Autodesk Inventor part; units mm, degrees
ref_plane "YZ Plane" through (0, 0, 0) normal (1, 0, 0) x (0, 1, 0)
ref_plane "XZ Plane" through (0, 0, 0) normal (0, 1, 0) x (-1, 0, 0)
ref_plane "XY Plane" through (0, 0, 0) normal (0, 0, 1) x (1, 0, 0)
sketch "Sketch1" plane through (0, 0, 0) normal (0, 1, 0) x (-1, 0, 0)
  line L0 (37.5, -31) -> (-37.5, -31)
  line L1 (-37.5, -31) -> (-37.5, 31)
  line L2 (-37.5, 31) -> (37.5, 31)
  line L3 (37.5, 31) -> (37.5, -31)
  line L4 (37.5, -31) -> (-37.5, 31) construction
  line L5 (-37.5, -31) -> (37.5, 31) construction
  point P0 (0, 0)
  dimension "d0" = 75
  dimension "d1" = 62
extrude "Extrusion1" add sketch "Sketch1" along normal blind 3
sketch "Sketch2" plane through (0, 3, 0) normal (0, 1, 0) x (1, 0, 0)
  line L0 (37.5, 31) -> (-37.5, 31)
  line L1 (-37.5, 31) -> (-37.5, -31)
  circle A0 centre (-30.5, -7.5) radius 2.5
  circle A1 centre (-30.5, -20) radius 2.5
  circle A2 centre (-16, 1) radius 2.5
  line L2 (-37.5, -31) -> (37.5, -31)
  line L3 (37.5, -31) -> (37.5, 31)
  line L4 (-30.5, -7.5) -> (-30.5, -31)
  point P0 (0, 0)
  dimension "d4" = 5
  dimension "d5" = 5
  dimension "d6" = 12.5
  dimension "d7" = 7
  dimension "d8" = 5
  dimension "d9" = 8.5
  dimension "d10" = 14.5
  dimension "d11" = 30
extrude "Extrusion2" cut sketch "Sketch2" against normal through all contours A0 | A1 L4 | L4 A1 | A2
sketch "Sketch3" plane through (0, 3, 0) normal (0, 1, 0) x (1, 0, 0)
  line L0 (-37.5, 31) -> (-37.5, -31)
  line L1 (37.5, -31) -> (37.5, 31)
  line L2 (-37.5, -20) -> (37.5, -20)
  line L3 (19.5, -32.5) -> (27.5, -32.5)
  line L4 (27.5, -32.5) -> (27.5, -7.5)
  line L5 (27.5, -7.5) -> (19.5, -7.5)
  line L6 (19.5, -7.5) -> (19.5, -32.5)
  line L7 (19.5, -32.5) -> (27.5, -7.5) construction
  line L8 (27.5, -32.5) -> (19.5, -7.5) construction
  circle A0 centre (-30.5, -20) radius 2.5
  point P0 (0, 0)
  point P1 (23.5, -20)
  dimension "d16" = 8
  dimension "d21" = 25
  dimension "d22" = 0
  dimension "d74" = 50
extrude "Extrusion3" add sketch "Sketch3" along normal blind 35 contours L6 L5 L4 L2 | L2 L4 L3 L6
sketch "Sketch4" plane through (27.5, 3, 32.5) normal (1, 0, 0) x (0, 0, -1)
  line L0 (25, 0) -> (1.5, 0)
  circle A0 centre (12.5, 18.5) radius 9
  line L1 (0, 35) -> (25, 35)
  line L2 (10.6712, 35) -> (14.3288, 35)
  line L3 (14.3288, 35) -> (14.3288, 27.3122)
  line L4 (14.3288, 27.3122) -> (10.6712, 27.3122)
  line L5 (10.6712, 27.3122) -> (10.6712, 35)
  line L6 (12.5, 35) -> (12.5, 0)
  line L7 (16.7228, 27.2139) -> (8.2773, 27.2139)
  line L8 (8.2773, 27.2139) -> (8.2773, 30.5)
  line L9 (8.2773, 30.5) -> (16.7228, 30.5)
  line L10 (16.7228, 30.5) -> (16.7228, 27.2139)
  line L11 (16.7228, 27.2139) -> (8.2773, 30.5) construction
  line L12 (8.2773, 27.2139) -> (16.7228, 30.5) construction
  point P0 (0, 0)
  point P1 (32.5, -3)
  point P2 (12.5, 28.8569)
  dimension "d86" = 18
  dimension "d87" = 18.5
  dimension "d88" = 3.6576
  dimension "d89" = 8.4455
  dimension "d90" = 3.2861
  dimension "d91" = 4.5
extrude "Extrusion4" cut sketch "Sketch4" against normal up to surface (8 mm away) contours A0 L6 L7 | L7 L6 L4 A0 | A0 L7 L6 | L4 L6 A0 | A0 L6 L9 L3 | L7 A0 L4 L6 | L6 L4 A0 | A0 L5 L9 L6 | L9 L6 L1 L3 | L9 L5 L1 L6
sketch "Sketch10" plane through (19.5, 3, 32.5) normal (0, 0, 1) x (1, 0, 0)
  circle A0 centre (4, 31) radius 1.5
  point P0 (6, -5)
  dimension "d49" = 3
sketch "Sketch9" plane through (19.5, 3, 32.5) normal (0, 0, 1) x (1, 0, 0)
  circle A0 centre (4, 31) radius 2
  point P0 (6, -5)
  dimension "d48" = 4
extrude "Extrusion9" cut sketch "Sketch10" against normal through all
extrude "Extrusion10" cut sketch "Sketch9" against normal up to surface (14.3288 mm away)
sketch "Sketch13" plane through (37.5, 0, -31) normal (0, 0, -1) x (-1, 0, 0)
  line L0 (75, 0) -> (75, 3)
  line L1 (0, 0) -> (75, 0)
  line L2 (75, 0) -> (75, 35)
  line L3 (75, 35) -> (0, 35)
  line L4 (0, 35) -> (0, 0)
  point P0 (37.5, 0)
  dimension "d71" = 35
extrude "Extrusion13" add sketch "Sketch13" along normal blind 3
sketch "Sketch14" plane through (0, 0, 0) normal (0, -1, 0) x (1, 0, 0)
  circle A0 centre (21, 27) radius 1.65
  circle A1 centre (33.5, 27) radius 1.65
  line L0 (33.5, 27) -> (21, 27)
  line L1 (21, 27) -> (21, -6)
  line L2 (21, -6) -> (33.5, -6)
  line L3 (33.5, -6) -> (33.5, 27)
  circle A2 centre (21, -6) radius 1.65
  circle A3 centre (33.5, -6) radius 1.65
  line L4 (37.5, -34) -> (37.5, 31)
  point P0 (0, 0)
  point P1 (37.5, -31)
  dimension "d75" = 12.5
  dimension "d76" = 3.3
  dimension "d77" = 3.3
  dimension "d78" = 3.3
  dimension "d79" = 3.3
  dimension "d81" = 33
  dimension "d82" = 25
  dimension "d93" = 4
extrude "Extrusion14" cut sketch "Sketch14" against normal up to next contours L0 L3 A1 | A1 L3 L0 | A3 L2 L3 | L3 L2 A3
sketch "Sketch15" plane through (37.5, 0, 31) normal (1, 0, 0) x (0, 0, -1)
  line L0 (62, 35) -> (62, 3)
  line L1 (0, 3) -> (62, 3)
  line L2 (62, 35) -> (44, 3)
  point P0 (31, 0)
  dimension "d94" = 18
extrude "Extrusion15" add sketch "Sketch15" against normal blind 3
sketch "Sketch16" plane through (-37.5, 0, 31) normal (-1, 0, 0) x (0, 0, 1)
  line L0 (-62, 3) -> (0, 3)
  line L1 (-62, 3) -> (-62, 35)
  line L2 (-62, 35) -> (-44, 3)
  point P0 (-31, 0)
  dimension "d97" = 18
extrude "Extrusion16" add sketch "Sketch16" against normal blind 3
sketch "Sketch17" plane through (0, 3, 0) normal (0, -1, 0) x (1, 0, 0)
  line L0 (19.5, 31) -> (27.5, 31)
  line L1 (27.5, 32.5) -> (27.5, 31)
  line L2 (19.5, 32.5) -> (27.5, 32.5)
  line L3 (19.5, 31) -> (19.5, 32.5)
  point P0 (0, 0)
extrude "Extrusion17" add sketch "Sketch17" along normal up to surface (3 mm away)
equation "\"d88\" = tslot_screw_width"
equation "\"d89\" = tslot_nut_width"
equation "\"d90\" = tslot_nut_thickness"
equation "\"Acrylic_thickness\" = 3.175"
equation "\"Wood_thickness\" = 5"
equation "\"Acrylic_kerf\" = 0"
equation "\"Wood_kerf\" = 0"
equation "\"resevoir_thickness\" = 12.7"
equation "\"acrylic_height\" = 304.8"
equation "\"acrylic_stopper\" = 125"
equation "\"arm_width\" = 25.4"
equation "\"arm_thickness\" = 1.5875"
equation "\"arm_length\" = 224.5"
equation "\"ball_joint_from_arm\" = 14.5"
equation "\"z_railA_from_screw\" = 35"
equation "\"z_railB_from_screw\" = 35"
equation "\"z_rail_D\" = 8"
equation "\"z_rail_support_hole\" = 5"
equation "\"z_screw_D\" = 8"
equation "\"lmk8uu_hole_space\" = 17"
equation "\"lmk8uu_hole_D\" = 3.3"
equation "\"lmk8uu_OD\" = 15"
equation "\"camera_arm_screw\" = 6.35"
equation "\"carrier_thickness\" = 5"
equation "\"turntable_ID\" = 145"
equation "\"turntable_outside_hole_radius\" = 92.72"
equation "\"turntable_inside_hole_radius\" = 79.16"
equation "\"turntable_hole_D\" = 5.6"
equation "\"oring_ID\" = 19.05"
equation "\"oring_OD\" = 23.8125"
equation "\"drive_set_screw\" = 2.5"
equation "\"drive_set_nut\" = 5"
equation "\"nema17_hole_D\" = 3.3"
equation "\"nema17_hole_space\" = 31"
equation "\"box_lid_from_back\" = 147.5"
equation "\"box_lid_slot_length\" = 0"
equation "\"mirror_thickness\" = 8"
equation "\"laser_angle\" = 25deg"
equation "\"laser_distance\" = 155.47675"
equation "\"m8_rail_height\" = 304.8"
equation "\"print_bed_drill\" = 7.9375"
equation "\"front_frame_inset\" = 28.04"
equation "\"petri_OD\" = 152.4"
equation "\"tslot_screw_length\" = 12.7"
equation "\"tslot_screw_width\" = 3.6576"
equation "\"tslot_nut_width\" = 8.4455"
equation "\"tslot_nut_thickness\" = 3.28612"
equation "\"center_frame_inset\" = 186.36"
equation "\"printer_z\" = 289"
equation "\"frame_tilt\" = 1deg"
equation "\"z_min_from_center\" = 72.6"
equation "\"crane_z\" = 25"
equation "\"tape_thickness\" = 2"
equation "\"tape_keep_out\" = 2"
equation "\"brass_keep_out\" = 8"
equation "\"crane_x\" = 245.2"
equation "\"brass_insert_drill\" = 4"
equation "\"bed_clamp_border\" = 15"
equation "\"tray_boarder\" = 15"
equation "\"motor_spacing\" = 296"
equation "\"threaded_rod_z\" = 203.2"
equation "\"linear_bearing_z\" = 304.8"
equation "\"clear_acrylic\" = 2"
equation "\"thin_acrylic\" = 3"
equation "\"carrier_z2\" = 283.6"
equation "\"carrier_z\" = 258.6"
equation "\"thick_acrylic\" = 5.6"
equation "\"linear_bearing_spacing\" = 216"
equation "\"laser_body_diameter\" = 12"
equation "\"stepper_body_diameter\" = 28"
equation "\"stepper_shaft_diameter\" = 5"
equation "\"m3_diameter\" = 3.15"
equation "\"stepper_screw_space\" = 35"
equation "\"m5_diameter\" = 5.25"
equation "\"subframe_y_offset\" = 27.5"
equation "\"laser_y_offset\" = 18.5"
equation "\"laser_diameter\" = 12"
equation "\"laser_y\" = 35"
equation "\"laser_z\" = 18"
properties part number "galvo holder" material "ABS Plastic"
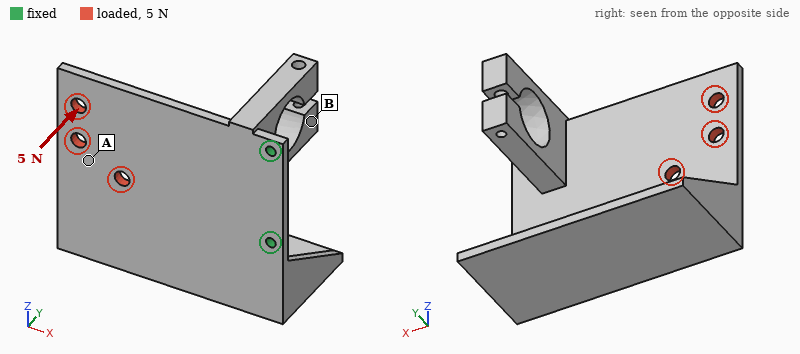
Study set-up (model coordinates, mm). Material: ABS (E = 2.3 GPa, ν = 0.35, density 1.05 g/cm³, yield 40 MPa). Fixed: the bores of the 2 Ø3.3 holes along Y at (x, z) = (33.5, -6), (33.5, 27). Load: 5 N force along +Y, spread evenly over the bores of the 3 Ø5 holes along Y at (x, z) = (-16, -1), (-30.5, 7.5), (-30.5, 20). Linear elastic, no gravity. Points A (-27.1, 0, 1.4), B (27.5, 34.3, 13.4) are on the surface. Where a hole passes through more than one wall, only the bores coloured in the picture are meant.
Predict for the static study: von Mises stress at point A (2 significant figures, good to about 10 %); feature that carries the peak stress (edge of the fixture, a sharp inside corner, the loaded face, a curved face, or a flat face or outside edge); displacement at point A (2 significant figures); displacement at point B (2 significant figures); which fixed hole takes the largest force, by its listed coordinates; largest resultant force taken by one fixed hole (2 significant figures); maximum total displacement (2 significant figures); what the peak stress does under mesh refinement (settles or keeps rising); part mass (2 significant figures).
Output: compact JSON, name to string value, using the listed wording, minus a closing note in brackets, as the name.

{"von Mises stress at point A": "1.1 MPa", "feature that carries the peak stress": "edge of the fixture", "displacement at point A": "0.91 mm", "displacement at point B": "0.31 mm", "which fixed hole takes the largest force, by its listed coordinates": "(33.5, -6)", "largest resultant force taken by one fixed hole": "4.1 N", "maximum total displacement": "1.2 mm", "what the peak stress does under mesh refinement": "keeps rising", "part mass": "29 g"}
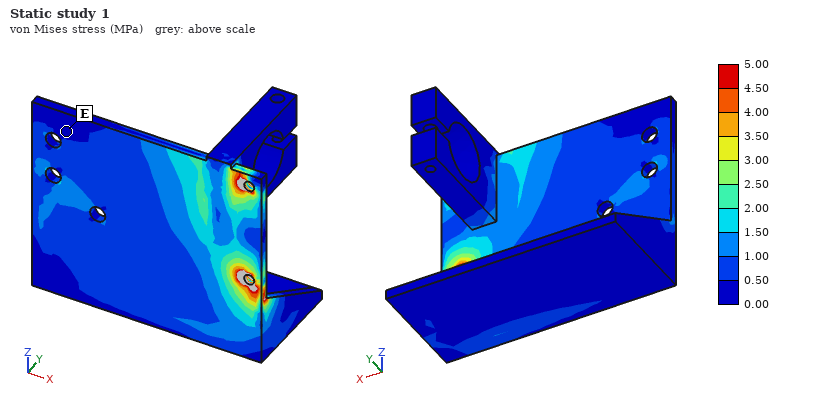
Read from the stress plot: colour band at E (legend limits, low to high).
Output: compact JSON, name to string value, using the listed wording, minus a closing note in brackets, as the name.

{"colour band at E": "0.00 to 0.50 MPa"}
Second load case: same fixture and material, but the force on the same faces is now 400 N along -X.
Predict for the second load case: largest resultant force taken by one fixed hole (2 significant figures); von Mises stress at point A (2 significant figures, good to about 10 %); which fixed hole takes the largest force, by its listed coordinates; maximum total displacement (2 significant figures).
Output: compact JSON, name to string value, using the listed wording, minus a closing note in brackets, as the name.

{"largest resultant force taken by one fixed hole": "220 N", "von Mises stress at point A": "1.5 MPa", "which fixed hole takes the largest force, by its listed coordinates": "(33.5, -6)", "maximum total displacement": "0.12 mm"}
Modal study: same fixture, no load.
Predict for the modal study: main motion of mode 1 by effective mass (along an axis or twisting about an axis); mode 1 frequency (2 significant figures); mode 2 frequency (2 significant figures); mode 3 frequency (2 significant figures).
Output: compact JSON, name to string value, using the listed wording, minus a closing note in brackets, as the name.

{"main motion of mode 1 by effective mass": "along Y", "mode 1 frequency": "110 Hz", "mode 2 frequency": "200 Hz", "mode 3 frequency": "410 Hz"}
